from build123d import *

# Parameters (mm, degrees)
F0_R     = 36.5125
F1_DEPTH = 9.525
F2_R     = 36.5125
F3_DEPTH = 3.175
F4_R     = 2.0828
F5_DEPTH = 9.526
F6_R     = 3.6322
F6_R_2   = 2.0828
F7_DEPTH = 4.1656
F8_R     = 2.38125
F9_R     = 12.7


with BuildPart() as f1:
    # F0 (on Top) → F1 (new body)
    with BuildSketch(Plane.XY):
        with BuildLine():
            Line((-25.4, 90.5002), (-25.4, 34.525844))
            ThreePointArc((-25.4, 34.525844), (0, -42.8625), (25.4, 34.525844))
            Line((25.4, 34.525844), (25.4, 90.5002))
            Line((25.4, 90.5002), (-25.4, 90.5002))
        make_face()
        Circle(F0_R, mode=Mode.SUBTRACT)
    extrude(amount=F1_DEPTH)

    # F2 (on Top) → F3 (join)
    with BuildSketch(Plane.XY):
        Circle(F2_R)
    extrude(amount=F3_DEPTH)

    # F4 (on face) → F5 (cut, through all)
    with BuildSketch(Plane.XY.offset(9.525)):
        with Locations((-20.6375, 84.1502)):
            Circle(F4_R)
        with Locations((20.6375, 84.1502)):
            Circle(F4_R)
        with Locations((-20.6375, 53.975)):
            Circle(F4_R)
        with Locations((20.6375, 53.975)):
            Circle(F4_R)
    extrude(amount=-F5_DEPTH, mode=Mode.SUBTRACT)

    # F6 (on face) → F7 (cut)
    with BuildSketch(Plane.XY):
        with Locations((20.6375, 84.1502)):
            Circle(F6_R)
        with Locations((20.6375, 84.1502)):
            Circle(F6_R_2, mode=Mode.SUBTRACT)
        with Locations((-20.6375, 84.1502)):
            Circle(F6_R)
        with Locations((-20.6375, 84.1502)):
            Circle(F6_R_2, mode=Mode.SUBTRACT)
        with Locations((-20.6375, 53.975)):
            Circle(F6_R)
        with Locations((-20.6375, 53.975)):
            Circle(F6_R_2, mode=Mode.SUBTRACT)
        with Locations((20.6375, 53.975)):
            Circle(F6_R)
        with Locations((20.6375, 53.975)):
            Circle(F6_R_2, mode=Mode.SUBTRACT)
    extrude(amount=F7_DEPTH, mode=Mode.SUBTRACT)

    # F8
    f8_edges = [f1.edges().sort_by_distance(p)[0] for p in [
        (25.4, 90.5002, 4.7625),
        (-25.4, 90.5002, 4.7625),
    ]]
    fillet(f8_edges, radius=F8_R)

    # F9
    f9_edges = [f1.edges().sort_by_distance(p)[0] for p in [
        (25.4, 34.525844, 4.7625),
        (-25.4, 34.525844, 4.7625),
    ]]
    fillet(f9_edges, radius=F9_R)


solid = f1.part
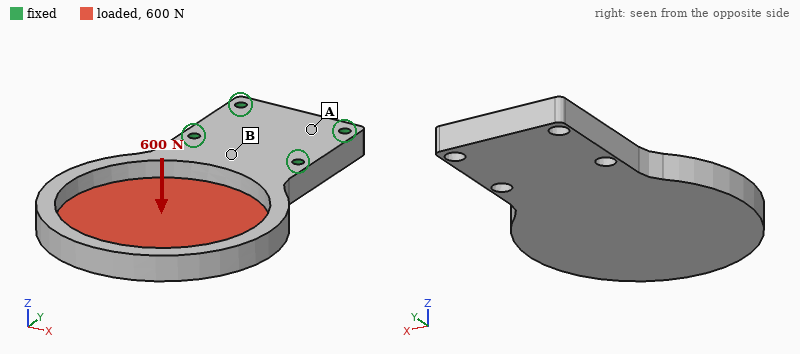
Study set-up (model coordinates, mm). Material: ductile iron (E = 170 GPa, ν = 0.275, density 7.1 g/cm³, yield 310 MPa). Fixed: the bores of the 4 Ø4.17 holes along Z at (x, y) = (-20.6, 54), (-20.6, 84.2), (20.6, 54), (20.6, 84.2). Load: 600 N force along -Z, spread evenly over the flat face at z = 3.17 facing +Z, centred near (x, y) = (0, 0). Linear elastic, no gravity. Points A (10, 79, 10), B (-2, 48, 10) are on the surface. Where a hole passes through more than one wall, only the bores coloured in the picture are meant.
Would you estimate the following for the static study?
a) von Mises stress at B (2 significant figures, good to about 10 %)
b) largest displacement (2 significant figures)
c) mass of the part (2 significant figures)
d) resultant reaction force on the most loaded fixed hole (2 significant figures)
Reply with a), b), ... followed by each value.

a) 22 MPa
b) 0.31 mm
c) 370 g
d) 860 N
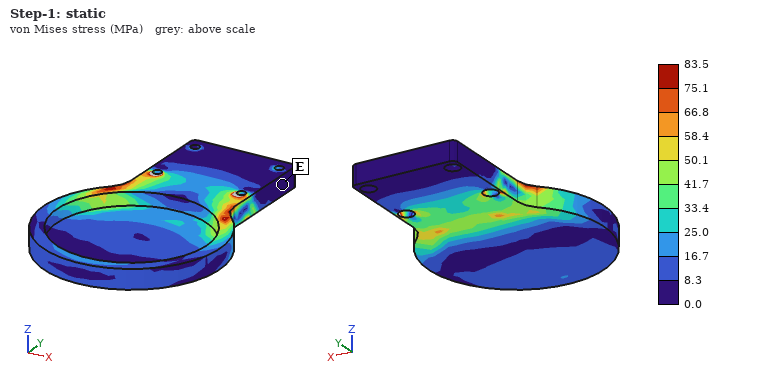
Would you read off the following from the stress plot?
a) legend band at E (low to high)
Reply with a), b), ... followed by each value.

a) 0.0 to 8.3 MPa
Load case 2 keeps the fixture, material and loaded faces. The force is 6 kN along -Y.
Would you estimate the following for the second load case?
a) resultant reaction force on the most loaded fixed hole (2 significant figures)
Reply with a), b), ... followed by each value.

a) 2.2 kN
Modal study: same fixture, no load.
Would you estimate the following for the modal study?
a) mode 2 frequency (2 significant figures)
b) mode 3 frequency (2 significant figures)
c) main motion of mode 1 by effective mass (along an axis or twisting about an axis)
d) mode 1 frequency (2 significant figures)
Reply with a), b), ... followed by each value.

a) 1500 Hz
b) 3100 Hz
c) along Z
d) 620 Hz
